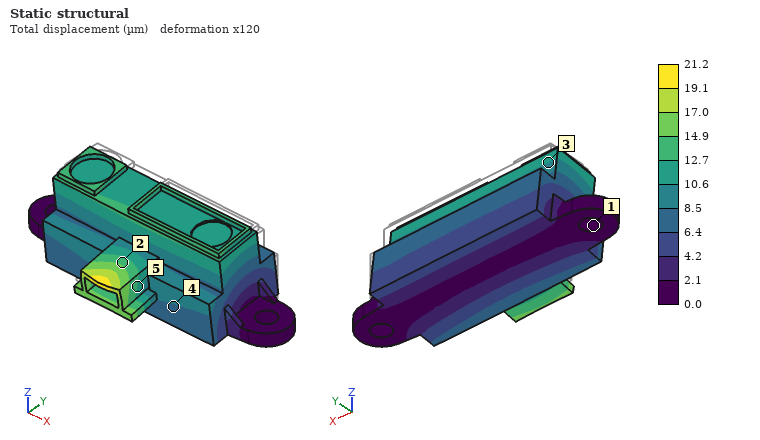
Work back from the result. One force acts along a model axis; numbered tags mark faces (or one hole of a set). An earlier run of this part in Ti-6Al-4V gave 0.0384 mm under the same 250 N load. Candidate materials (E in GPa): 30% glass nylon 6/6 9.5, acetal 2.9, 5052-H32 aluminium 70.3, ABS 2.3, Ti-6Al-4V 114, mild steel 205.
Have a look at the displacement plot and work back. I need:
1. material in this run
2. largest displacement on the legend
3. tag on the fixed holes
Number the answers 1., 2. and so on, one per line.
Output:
1. mild steel
2. 21.2 µm
3. 1
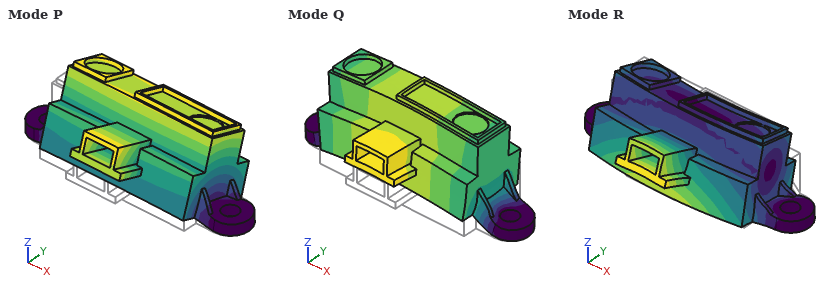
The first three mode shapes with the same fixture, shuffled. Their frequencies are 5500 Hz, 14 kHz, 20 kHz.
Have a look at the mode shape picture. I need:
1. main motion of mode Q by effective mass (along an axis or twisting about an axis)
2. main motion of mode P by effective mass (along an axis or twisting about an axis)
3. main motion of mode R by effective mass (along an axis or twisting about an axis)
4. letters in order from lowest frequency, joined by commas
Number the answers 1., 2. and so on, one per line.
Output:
1. along Z
2. along Y
3. along Y
4. P, Q, R
